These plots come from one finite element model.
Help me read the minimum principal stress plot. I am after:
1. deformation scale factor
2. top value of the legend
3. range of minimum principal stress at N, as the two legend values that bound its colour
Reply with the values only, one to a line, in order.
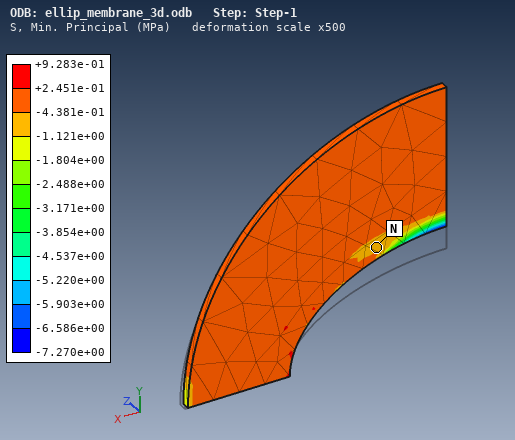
500
+9.283e-01 MPa
-1.121e+00 to -4.381e-01 MPa
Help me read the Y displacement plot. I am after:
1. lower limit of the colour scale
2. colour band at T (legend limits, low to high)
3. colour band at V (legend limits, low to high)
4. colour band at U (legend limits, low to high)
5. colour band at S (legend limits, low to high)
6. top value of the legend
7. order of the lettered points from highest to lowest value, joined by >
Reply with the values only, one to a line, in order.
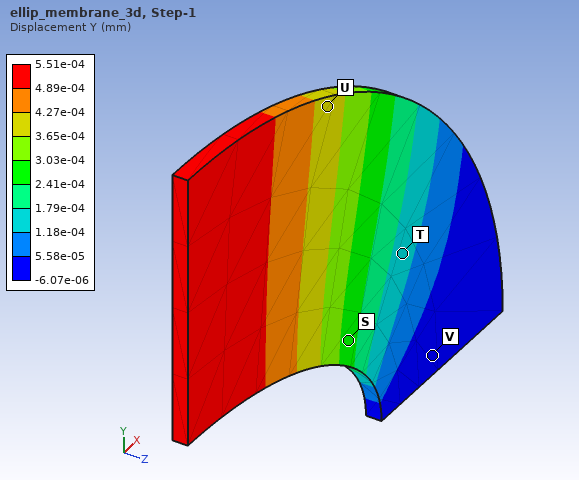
-6.07e-06 mm
1.18e-04 to 1.79e-04 mm
-6.07e-06 to 5.58e-05 mm
3.65e-04 to 4.27e-04 mm
2.41e-04 to 3.03e-04 mm
5.51e-04 mm
U > S > T > V
